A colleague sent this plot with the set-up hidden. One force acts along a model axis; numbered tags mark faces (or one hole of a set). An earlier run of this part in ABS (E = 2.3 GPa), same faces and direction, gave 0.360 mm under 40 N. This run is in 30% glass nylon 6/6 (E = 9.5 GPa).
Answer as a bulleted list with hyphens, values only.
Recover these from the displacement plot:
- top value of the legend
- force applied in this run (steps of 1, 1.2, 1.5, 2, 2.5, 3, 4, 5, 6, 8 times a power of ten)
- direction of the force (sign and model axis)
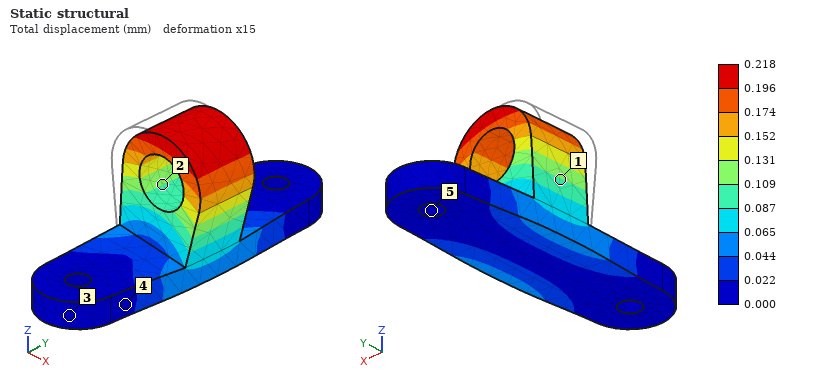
- 0.218 mm
- 100 N
- +X
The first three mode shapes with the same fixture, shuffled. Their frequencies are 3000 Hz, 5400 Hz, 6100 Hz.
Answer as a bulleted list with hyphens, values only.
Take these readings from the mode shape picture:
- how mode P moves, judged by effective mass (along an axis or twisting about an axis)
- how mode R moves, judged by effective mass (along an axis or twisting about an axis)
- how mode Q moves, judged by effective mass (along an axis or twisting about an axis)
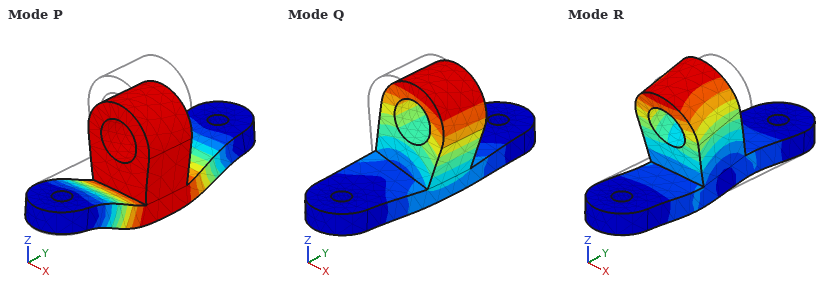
- along Z
- along Y
- along X
